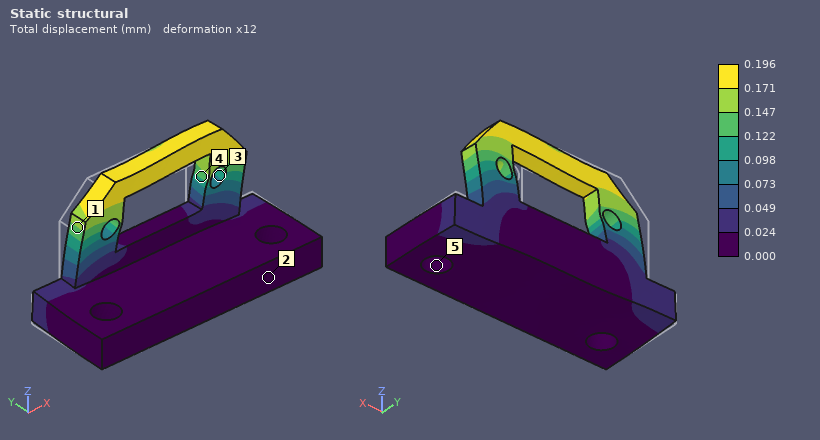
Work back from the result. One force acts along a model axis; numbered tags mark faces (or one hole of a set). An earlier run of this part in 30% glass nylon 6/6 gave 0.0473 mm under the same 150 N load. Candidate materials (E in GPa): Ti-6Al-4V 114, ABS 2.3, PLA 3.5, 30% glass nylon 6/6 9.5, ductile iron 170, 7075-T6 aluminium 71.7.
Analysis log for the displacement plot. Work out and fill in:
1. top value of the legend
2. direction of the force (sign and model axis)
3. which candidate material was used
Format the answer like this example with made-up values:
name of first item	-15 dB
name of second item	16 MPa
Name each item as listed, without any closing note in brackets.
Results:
top value of the legend	0.196 mm
direction of the force	+X
which candidate material was used	ABS
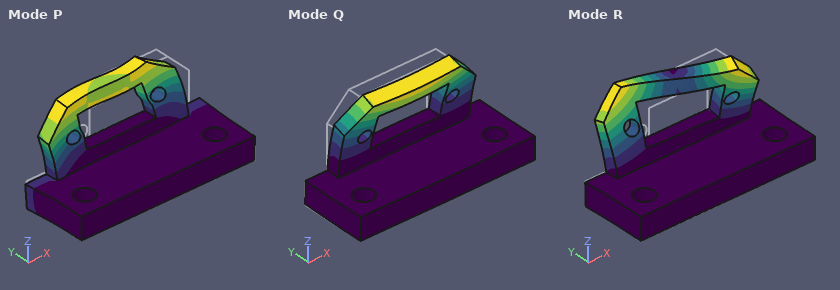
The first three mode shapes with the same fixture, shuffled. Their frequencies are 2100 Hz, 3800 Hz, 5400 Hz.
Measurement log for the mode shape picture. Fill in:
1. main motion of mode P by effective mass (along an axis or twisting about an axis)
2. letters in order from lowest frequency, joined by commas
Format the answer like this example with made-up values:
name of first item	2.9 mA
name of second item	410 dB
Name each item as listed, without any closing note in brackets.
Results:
main motion of mode P by effective mass	along X
letters in order from lowest frequency, joined by commas	Q, R, P
